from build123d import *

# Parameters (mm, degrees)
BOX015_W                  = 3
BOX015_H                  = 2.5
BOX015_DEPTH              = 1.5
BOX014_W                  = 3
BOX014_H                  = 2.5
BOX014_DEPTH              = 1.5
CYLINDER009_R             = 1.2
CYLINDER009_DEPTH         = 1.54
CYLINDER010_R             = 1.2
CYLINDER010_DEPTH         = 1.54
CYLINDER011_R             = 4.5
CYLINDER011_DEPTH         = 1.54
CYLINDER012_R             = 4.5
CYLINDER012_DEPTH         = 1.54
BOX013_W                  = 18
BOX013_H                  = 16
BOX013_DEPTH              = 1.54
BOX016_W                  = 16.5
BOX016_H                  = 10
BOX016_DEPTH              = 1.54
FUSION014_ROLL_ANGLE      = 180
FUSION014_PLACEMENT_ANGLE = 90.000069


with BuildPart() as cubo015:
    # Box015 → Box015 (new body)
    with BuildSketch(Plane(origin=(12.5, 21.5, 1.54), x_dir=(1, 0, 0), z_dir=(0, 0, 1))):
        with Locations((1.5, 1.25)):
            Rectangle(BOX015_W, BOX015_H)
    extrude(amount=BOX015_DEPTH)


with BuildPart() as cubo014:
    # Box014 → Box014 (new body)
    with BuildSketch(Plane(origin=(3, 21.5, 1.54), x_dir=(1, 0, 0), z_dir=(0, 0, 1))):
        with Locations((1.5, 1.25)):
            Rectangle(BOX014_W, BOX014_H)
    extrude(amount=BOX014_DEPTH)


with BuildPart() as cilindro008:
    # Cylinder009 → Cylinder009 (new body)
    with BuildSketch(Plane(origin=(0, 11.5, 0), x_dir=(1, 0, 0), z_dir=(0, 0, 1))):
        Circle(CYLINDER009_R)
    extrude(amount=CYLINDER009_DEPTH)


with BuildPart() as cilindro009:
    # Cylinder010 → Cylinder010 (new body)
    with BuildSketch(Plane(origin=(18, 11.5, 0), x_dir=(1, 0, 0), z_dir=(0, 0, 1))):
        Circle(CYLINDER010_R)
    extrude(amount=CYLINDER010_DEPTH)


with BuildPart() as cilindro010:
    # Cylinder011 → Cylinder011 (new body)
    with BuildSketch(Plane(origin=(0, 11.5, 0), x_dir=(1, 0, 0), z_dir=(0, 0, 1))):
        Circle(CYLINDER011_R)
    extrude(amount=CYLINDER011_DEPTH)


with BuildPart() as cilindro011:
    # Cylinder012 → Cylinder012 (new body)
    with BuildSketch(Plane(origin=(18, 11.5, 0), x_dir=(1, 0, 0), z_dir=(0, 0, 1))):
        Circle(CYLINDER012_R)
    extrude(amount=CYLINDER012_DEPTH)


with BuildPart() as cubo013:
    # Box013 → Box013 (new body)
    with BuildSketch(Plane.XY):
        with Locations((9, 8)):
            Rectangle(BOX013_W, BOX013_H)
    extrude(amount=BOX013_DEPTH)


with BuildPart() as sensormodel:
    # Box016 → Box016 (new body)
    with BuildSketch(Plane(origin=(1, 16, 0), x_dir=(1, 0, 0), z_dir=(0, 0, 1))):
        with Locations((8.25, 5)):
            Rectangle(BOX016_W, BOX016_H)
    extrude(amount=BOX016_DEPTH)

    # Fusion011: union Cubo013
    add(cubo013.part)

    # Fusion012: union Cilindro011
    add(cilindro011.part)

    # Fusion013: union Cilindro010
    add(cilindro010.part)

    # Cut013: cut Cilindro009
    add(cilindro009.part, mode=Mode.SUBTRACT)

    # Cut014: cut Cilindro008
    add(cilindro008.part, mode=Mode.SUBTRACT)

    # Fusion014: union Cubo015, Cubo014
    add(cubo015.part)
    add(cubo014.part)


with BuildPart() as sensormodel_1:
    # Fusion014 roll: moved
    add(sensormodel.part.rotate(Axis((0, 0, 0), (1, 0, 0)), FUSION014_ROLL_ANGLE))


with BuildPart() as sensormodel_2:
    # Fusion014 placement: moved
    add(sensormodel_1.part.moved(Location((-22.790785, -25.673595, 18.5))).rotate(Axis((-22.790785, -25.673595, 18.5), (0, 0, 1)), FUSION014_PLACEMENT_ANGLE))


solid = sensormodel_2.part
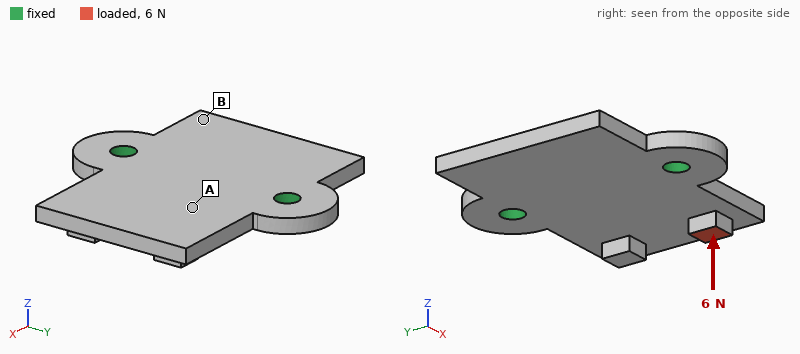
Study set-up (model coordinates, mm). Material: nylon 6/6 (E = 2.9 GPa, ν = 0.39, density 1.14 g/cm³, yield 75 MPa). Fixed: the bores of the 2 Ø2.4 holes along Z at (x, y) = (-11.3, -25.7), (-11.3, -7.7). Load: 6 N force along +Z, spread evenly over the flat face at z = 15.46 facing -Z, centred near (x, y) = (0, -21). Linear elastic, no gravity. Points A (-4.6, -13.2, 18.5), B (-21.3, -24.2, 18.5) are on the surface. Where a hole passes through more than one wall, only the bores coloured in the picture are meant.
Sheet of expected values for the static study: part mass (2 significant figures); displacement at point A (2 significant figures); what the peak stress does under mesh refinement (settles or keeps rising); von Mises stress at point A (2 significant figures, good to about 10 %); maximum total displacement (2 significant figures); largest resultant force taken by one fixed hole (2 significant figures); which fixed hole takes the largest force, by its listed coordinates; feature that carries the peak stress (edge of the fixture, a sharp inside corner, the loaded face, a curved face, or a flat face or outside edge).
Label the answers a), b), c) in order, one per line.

a) 0.92 g
b) 0.086 mm
c) keeps rising
d) 4.1 MPa
e) 0.35 mm
f) 4.8 N
g) (-11.3, -25.7)
h) edge of the fixture
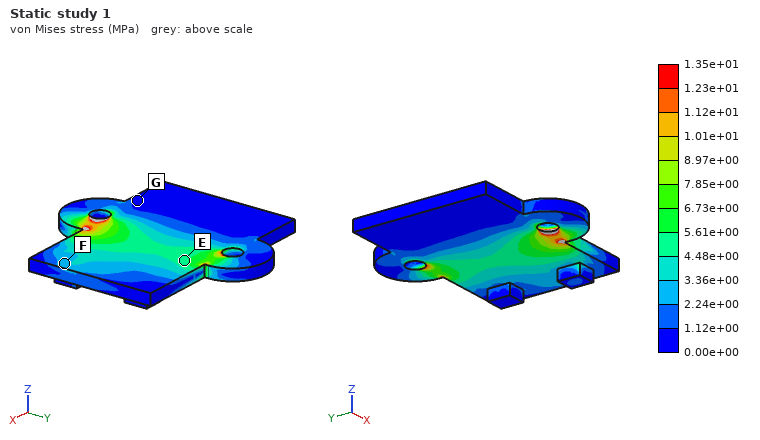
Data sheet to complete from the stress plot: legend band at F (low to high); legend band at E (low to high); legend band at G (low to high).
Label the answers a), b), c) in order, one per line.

a) 2.24e+00 to 3.36e+00 MPa
b) 4.48e+00 to 5.61e+00 MPa
c) 0.00e+00 to 1.12e+00 MPa
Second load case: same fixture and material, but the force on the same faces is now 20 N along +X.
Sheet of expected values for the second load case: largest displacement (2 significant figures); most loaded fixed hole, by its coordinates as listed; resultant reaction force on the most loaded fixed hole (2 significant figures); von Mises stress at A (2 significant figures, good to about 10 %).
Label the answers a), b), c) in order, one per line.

a) 0.36 mm
b) (-11.3, -25.7)
c) 15 N
d) 5.4 MPa
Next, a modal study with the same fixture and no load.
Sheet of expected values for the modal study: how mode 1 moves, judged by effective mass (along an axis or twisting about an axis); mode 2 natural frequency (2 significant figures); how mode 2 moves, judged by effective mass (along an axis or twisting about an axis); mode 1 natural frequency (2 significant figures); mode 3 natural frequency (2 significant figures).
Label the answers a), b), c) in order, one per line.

a) along Z
b) 3000 Hz
c) along Z
d) 1700 Hz
e) 4400 Hz
